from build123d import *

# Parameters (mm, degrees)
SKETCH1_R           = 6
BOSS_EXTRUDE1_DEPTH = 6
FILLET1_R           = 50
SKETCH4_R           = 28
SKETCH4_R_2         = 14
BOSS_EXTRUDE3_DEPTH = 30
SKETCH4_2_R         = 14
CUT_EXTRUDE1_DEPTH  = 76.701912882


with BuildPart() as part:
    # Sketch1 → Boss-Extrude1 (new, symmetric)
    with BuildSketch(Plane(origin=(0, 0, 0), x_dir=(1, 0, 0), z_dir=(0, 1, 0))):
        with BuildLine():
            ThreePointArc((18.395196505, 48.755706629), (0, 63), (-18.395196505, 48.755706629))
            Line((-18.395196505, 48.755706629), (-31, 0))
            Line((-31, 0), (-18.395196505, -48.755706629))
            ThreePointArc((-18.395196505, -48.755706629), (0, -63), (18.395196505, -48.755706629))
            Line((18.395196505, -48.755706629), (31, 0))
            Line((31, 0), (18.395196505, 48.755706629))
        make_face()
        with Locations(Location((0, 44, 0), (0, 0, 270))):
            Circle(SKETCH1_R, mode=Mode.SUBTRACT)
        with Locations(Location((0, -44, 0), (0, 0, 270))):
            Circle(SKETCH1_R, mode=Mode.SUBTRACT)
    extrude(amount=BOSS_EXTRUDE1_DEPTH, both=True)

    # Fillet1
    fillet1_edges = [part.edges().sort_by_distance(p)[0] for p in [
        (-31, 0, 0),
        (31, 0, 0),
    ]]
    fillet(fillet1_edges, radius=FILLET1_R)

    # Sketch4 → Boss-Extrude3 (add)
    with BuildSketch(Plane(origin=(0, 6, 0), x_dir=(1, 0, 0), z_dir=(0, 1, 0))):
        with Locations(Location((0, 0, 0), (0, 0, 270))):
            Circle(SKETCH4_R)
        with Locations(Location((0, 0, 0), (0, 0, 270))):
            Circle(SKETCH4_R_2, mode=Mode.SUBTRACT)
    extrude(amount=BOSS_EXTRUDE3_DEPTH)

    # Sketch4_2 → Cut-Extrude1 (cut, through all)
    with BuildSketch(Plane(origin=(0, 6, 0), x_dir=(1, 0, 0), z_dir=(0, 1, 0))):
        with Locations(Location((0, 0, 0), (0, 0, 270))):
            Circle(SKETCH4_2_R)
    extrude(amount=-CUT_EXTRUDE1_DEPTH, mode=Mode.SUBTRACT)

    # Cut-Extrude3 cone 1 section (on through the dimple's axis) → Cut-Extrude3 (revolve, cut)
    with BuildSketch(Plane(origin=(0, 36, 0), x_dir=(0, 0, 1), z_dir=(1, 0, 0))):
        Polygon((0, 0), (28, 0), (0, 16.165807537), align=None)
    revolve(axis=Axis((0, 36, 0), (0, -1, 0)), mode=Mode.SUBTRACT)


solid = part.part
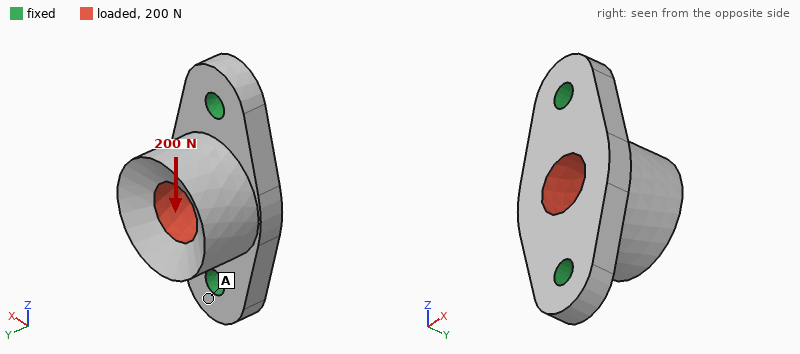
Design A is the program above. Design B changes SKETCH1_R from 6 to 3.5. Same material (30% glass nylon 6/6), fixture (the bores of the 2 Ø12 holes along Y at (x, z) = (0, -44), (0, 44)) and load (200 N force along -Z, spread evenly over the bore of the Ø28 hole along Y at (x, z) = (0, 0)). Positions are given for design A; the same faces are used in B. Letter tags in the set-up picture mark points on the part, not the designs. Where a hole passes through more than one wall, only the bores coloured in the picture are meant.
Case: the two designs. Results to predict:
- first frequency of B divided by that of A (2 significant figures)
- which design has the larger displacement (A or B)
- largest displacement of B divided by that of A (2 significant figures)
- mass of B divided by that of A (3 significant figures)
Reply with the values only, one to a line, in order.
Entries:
0.85
B
1.2
1.02
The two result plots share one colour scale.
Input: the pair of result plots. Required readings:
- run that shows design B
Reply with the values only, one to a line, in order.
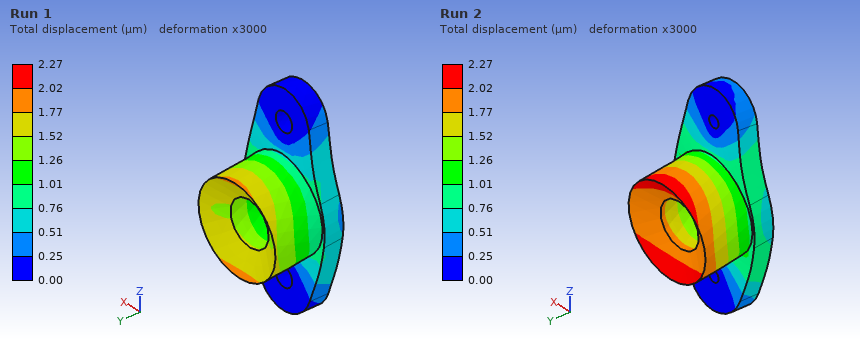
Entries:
Run 2
